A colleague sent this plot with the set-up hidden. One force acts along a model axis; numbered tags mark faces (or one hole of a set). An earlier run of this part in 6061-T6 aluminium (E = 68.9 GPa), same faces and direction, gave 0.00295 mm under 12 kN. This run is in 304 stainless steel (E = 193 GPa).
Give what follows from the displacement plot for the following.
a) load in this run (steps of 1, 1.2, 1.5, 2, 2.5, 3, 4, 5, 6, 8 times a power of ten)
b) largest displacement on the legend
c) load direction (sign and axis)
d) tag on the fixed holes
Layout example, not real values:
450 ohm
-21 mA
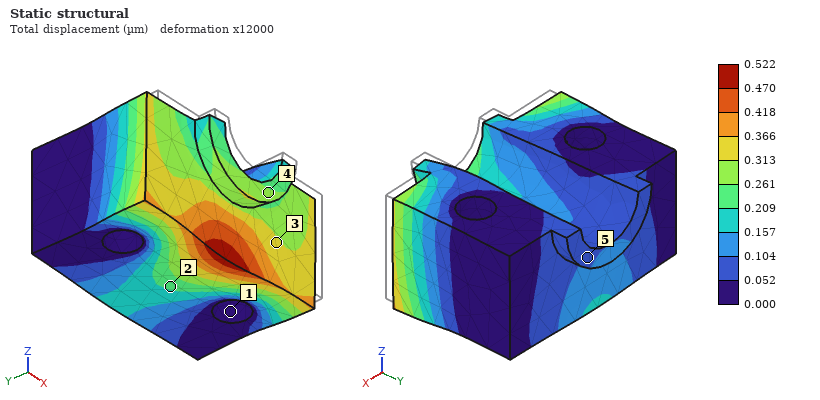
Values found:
6 kN
0.522 µm
+Y
1
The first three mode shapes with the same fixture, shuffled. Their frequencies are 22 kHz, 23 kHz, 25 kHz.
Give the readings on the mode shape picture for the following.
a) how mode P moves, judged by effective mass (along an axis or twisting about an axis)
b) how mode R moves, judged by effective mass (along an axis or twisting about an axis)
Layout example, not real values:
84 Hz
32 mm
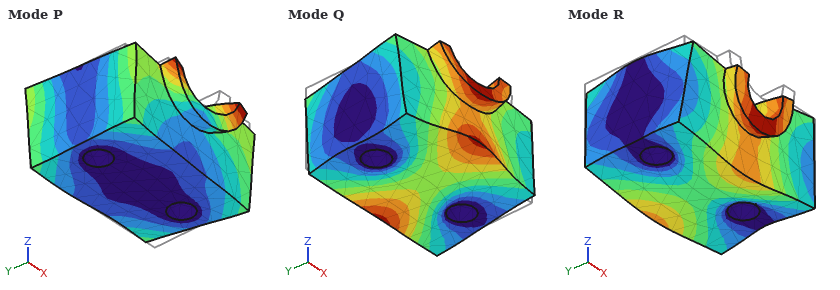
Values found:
twisting about Z
along Z
